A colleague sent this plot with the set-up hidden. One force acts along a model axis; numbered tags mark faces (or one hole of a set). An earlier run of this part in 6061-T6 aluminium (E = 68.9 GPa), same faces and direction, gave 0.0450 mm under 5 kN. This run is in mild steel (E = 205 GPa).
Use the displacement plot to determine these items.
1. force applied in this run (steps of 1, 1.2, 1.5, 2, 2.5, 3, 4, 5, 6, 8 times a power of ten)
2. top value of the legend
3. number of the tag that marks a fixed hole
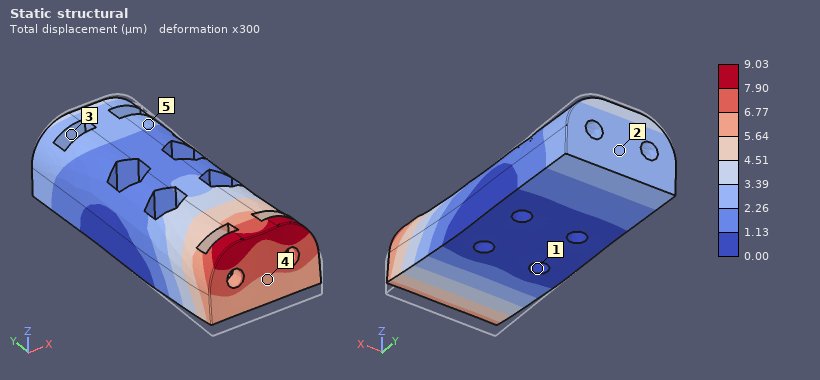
3 kN
9.03 µm
1
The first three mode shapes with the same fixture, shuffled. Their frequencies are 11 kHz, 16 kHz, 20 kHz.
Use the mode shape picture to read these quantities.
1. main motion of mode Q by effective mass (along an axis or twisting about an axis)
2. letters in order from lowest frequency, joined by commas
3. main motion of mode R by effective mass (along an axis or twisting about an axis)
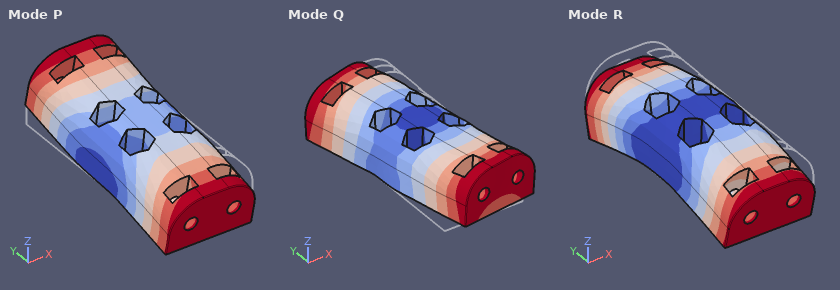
twisting about Z
P, R, Q
along Z
